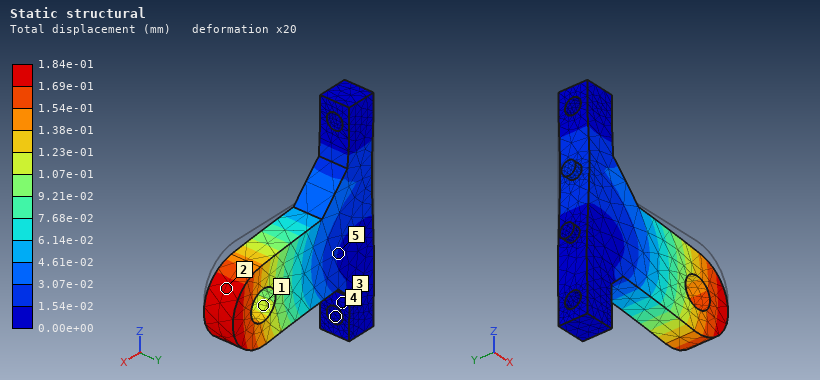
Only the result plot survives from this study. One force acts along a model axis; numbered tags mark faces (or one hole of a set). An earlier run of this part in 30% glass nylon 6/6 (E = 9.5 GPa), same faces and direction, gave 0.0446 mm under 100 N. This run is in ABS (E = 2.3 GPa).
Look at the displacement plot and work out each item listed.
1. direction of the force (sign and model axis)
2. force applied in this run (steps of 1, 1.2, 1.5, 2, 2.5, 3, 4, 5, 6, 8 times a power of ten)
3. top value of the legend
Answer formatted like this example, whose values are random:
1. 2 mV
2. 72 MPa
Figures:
1. -Z
2. 100 N
3. 1.84e-01 mm
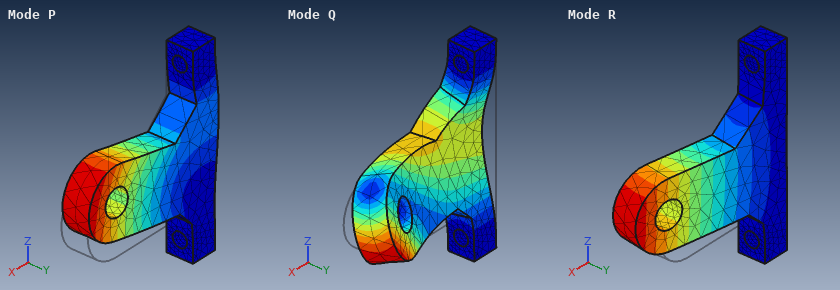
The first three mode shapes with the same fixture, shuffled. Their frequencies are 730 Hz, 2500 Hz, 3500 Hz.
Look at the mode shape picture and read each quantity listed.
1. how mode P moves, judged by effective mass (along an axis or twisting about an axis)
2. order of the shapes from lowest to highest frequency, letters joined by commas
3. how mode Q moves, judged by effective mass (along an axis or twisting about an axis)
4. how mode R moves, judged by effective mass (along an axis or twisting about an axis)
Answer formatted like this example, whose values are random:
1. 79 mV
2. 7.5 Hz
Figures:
1. along Z
2. R, P, Q
3. along Y
4. along Y
